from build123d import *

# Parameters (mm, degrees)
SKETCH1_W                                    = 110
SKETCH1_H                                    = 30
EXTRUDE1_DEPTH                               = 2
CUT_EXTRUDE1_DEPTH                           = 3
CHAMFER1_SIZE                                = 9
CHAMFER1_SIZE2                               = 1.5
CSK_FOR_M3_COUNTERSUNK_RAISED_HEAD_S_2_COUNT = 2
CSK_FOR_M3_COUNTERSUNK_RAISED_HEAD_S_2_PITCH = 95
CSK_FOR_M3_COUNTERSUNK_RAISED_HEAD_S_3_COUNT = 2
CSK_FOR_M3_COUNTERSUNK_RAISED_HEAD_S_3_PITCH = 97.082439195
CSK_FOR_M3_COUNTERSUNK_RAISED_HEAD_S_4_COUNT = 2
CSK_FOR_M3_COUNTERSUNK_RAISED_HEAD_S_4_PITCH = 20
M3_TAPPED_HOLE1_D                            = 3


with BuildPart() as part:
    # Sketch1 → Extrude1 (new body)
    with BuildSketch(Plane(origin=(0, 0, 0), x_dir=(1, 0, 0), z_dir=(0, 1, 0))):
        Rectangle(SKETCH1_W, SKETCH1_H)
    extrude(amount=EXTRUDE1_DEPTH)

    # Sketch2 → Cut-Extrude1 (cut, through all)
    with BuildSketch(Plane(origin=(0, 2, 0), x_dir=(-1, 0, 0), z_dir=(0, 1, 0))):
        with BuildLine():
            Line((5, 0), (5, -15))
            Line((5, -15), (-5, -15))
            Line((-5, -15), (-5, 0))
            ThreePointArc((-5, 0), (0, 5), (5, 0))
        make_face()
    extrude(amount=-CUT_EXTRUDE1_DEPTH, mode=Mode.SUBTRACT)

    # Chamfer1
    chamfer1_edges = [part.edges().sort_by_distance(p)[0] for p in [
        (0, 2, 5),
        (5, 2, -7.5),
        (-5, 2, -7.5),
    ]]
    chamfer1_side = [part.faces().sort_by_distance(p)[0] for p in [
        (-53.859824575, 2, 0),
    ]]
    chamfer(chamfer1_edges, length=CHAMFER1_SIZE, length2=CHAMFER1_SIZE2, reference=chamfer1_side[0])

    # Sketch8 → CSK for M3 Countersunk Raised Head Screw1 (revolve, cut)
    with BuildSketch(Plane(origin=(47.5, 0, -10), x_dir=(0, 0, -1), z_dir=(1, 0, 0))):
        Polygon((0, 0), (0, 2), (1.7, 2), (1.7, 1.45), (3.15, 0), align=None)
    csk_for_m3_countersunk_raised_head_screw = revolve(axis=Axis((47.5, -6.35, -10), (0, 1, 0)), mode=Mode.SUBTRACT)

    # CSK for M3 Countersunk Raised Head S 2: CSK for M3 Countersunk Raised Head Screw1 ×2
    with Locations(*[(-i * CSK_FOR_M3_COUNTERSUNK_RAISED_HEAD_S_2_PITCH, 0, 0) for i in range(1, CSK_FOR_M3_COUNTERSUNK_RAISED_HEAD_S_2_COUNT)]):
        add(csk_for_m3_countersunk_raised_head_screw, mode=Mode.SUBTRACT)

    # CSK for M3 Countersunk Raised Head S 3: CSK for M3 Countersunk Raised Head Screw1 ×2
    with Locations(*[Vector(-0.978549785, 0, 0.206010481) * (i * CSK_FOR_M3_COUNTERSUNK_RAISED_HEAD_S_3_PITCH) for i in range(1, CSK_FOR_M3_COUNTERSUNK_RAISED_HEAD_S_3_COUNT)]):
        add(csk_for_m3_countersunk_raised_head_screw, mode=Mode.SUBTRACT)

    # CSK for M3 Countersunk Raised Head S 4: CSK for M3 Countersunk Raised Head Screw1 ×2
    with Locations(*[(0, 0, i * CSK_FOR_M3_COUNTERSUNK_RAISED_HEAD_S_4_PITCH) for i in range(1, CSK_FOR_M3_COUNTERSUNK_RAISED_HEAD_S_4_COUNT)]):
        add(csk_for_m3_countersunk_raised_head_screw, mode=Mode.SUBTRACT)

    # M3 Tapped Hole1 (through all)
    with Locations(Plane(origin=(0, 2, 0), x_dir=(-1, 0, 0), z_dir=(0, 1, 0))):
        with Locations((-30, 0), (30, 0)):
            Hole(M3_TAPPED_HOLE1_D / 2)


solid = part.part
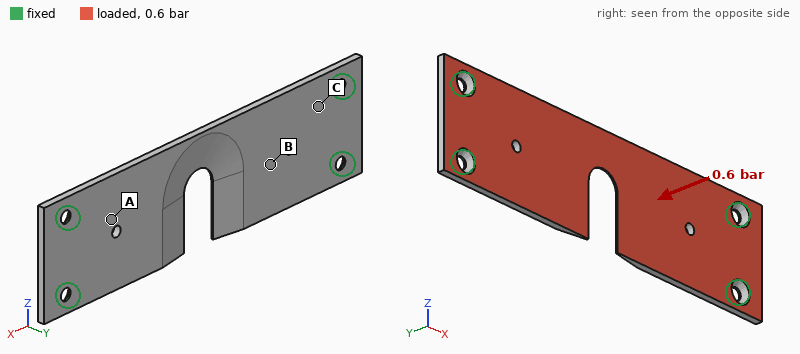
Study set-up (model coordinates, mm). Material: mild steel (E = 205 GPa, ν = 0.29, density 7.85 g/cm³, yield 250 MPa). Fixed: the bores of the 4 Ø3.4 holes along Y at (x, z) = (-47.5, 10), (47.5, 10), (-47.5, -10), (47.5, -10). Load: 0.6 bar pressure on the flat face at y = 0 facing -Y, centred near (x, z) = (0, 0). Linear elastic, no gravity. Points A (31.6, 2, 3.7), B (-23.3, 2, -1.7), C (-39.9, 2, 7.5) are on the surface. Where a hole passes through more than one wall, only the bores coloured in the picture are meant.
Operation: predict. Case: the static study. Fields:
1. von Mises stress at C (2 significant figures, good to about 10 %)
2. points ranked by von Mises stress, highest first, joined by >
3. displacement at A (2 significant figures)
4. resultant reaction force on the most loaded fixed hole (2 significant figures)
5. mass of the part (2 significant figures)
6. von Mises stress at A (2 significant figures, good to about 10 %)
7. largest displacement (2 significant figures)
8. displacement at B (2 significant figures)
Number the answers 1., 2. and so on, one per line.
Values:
1. 45 MPa
2. C > A > B
3. 0.050 mm
4. 180 N
5. 45 g
6. 25 MPa
7. 0.18 mm
8. 0.089 mm
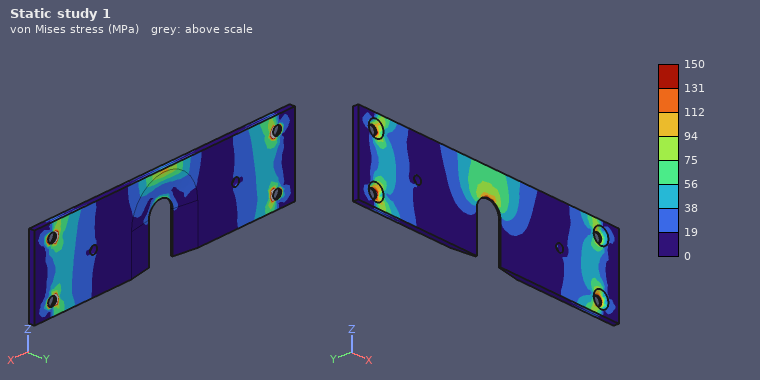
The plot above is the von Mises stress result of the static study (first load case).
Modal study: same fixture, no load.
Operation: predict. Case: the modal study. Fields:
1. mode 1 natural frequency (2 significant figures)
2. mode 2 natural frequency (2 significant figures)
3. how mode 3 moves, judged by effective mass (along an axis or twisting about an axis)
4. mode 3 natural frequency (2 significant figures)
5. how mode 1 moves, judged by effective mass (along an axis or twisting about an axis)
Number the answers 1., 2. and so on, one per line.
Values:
1. 1000 Hz
2. 2000 Hz
3. twisting about X
4. 2800 Hz
5. along Y
